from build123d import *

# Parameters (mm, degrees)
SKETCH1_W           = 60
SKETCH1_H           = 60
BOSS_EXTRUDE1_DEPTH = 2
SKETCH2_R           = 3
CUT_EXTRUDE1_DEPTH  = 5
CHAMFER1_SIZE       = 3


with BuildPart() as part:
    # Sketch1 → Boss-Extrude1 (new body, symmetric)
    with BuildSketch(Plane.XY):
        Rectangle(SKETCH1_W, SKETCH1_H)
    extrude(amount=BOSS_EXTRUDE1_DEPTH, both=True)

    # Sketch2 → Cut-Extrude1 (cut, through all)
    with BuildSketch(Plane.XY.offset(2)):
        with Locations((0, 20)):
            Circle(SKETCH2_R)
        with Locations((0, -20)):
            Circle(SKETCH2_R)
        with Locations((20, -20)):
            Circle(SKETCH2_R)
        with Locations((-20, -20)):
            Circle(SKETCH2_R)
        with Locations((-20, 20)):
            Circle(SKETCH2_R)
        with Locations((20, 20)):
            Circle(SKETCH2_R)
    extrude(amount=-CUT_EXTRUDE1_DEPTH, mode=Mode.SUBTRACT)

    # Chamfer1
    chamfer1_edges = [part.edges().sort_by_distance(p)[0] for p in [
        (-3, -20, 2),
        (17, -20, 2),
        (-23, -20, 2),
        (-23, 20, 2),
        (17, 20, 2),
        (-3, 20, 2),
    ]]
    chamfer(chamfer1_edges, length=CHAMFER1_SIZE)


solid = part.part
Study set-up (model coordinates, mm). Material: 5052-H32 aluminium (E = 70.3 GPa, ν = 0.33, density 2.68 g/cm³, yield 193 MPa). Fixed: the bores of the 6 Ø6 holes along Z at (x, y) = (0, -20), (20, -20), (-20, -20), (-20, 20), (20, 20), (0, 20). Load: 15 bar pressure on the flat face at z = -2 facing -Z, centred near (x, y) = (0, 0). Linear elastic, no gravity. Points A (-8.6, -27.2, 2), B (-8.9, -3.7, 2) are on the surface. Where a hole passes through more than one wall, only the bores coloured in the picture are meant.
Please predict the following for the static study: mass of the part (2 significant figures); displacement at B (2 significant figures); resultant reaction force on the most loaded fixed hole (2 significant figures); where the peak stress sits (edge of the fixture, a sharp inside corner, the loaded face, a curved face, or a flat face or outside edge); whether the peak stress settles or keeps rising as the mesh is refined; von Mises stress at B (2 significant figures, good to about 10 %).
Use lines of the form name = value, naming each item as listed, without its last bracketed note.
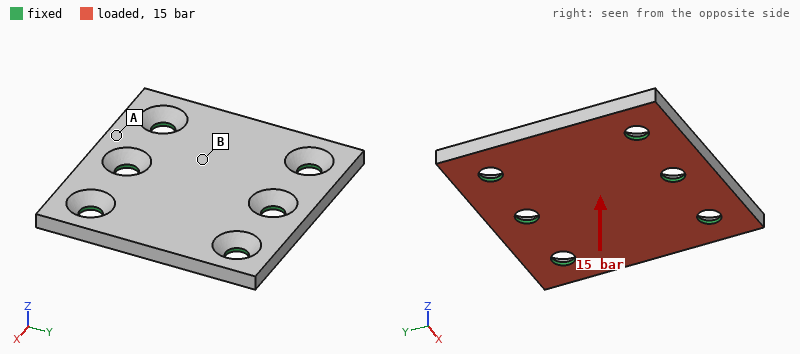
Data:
mass of the part = 35 g
displacement at B = 33 µm
resultant reaction force on the most loaded fixed hole = 1.1 kN
where the peak stress sits = edge of the fixture
whether the peak stress settles or keeps rising as the mesh is refined = keeps rising
von Mises stress at B = 40 MPa
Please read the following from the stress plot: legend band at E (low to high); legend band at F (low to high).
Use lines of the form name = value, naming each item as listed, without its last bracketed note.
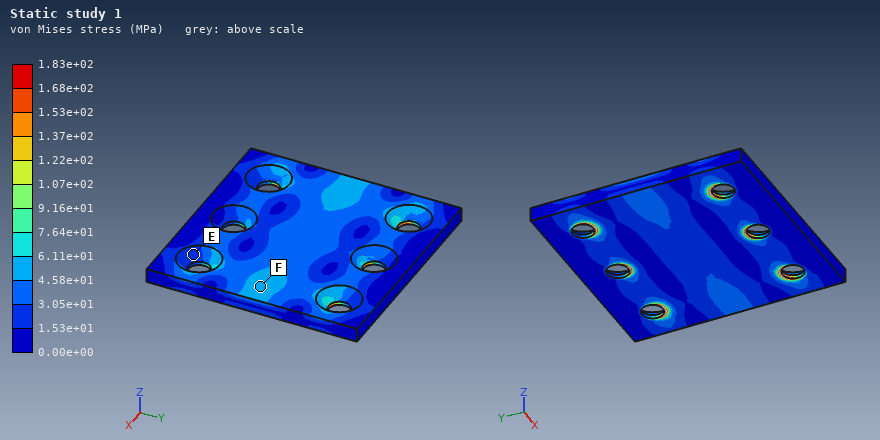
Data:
legend band at E = 1.53e+01 to 3.05e+01 MPa
legend band at F = 4.58e+01 to 6.11e+01 MPa
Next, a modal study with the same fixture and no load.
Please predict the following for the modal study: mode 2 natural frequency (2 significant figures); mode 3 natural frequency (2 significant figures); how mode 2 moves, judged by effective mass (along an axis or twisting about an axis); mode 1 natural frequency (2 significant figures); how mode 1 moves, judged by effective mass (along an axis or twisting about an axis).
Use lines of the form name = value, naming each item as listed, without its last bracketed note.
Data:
mode 2 natural frequency = 11 kHz
mode 3 natural frequency = 14 kHz
how mode 2 moves, judged by effective mass = twisting about Y
mode 1 natural frequency = 10 kHz
how mode 1 moves, judged by effective mass = along Z
